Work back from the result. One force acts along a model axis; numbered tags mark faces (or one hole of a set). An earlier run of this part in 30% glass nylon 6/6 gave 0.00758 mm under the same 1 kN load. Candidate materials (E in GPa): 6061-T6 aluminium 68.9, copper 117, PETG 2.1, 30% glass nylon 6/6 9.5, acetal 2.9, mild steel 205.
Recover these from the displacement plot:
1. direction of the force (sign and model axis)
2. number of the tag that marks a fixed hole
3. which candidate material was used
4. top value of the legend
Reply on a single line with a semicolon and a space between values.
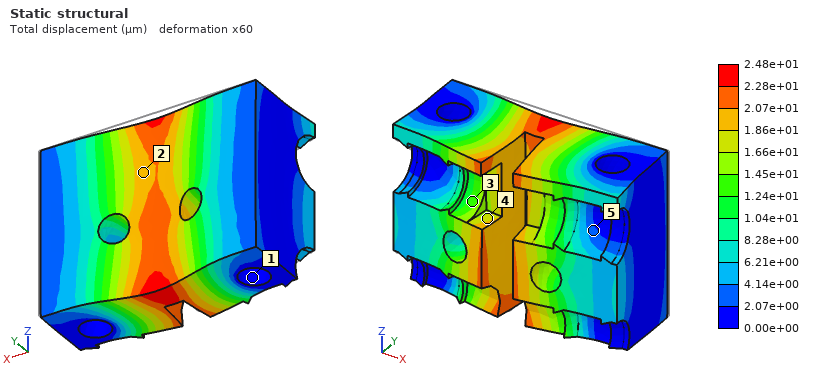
-Y; 1; acetal; 2.48e+01 µm
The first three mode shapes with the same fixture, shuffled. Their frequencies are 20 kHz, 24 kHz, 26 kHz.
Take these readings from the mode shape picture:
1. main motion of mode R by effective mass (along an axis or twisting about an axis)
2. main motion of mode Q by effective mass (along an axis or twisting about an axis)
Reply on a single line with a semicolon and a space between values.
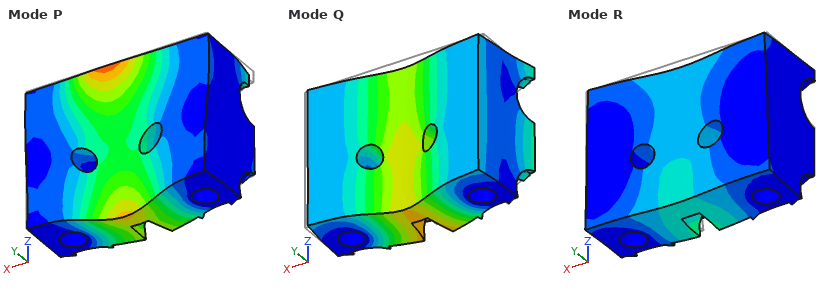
along Z; along Y
